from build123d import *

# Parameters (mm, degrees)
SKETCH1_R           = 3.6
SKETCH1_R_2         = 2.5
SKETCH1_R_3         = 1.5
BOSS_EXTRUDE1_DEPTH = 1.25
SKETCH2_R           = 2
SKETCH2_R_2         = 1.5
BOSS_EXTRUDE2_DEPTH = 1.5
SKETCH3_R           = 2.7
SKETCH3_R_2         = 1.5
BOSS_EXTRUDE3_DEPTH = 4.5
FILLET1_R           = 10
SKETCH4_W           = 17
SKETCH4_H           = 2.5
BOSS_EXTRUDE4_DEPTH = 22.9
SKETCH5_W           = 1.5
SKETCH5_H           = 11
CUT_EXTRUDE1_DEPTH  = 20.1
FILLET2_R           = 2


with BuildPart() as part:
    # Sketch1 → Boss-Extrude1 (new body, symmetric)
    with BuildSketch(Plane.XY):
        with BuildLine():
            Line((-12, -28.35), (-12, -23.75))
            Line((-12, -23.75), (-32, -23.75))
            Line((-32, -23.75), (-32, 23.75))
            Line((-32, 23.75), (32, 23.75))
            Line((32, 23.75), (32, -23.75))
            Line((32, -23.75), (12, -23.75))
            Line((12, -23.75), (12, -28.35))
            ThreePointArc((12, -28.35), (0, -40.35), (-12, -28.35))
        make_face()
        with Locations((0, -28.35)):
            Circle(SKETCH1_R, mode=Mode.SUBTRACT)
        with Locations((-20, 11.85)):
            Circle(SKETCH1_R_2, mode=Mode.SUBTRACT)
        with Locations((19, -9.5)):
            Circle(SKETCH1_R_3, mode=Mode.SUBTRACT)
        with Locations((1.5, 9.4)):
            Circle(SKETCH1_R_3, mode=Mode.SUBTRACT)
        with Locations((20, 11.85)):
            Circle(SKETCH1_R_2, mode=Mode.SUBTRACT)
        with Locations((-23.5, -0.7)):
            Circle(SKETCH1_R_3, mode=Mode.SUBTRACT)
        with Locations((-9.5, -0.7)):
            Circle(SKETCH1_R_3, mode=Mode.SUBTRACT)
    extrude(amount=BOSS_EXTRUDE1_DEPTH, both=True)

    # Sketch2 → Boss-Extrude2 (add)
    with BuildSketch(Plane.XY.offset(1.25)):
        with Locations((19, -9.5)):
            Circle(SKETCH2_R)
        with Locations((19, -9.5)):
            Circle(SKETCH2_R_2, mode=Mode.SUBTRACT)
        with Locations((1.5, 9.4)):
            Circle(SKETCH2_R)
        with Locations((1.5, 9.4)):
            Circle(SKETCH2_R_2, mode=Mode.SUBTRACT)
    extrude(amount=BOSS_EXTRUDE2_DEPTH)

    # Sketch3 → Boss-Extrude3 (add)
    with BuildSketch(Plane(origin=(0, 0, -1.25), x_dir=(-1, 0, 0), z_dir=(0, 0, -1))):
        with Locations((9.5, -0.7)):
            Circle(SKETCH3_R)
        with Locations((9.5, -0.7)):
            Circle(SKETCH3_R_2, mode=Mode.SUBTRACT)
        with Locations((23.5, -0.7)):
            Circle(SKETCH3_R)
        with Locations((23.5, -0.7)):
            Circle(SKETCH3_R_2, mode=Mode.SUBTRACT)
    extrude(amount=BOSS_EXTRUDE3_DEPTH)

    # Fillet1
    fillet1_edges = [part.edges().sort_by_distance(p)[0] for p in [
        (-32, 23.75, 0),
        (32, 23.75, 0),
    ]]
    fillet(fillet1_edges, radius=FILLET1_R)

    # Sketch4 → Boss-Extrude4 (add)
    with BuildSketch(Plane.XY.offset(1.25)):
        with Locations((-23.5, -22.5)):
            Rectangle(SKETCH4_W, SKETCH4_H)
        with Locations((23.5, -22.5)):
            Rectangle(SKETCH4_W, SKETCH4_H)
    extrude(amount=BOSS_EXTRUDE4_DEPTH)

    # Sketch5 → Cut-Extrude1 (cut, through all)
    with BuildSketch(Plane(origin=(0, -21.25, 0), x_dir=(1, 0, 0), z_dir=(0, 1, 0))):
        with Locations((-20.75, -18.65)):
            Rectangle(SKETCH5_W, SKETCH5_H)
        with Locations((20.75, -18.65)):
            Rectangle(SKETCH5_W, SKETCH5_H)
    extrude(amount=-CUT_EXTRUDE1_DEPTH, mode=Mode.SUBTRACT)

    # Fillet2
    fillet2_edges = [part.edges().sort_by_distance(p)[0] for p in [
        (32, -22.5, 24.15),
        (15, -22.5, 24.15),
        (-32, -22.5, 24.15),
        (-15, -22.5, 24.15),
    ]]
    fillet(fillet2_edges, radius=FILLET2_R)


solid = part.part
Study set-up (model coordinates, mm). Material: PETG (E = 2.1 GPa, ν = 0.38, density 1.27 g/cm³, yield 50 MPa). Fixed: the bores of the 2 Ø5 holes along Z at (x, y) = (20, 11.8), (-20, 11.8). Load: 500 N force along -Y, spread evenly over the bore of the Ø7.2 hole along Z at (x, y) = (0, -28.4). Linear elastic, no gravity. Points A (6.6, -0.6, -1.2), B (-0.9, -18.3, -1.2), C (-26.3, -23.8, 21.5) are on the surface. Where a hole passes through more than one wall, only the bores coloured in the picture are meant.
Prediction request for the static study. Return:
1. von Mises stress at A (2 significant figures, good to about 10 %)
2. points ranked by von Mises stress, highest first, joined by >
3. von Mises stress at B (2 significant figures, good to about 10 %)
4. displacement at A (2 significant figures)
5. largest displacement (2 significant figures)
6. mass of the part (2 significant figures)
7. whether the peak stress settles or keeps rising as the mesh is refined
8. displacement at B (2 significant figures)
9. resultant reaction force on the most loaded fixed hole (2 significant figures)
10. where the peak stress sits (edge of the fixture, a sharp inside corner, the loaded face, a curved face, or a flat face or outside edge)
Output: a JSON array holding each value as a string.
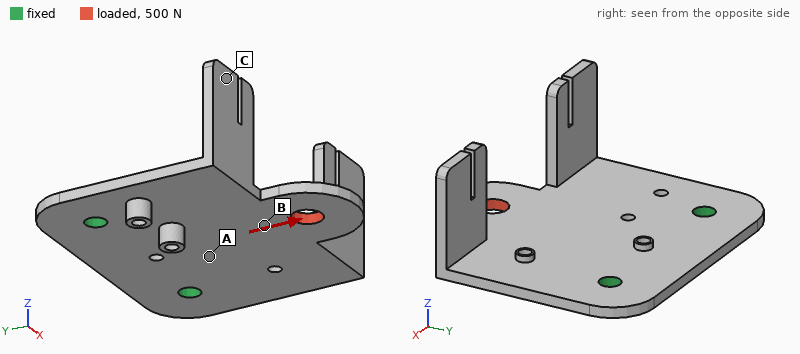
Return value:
["4.1 MPa", "B > A > C", "7.4 MPa", "0.052 mm", "0.17 mm", "13 g", "keeps rising", "0.10 mm", "260 N", "a sharp inside corner"]
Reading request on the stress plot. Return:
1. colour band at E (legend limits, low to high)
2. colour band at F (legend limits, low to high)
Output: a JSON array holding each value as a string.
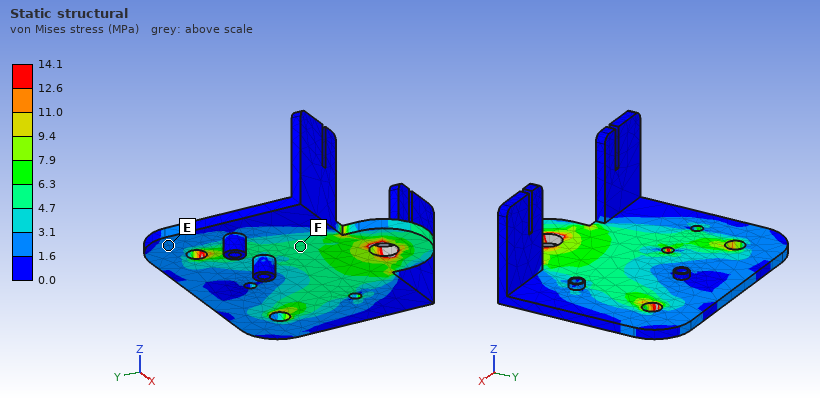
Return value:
["1.6 to 3.1 MPa", "4.7 to 6.3 MPa"]
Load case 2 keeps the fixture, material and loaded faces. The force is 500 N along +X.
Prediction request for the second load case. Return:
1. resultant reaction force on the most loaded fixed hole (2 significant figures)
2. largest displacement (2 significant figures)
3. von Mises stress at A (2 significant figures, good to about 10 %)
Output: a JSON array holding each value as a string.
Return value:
["530 N", "0.57 mm", "7.9 MPa"]
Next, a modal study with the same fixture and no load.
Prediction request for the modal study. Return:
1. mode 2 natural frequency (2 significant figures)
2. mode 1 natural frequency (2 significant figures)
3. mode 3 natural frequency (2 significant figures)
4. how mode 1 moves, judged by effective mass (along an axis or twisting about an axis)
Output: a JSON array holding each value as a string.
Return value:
["350 Hz", "220 Hz", "540 Hz", "along Z"]
